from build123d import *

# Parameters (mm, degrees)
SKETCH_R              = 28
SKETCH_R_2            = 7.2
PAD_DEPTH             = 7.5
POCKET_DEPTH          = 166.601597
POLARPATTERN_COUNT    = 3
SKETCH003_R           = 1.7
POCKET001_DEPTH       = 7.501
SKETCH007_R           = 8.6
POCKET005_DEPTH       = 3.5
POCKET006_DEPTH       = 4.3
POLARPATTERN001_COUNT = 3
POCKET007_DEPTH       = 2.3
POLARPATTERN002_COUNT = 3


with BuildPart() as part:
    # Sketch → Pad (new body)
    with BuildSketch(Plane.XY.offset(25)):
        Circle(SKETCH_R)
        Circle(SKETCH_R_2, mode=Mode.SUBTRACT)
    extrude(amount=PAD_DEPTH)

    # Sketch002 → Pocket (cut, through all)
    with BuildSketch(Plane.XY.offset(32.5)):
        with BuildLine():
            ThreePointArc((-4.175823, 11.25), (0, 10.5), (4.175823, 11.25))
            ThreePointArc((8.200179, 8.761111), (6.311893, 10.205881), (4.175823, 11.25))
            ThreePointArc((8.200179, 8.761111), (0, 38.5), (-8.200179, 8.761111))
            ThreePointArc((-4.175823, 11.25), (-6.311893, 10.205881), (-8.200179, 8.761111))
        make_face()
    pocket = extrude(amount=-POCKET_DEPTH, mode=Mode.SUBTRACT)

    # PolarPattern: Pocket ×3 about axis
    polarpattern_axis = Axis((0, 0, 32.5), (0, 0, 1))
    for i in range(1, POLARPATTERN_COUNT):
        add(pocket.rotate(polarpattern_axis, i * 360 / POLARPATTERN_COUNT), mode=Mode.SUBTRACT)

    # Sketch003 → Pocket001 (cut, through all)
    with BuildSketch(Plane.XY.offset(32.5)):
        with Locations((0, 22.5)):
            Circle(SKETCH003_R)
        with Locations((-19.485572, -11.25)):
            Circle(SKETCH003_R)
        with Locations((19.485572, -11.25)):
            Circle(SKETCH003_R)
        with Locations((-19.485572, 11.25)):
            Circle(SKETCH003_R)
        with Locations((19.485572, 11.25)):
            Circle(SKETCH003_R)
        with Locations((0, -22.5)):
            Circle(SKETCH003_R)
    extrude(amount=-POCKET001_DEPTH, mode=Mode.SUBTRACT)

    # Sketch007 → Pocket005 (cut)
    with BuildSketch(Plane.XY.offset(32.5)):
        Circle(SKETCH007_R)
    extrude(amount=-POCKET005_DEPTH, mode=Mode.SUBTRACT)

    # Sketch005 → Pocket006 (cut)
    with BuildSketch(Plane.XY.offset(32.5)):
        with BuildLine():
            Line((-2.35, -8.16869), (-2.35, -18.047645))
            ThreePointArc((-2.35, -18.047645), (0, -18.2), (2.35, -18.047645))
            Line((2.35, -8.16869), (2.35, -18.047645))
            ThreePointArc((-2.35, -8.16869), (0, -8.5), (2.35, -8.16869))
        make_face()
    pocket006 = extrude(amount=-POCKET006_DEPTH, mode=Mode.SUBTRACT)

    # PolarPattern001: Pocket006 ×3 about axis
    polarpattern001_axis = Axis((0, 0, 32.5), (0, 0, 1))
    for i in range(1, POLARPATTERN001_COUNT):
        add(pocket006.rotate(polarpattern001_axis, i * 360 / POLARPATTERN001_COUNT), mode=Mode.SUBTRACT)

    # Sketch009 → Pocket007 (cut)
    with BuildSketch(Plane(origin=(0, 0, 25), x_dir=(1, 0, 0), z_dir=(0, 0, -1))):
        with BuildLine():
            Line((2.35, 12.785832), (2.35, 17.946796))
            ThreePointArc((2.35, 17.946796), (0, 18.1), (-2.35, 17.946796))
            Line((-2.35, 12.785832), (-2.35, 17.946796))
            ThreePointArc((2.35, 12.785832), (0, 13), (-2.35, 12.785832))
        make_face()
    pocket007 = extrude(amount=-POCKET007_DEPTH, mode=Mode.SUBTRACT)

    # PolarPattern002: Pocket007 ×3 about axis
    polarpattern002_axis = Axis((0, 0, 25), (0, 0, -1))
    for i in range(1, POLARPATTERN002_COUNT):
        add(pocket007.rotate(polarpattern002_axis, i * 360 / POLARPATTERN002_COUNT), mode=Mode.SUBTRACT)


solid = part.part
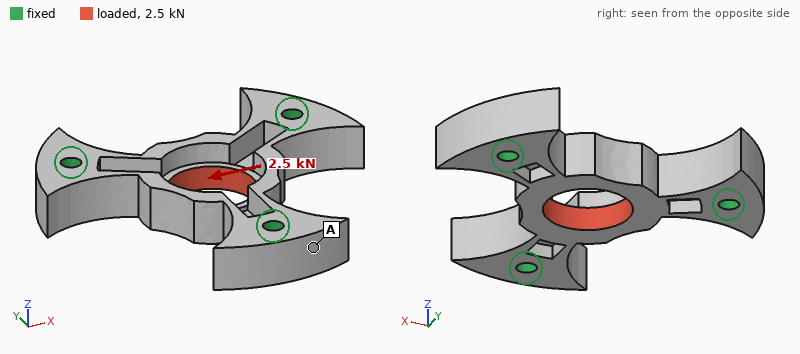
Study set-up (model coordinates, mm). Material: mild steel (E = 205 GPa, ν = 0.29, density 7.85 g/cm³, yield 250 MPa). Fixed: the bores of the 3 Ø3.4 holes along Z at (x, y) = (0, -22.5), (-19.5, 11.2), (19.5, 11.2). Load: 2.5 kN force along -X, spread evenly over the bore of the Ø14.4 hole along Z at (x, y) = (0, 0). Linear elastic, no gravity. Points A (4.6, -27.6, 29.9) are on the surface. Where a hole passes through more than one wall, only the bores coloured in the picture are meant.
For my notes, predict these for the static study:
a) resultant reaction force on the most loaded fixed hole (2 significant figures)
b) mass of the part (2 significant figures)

1.1 kN
42 g
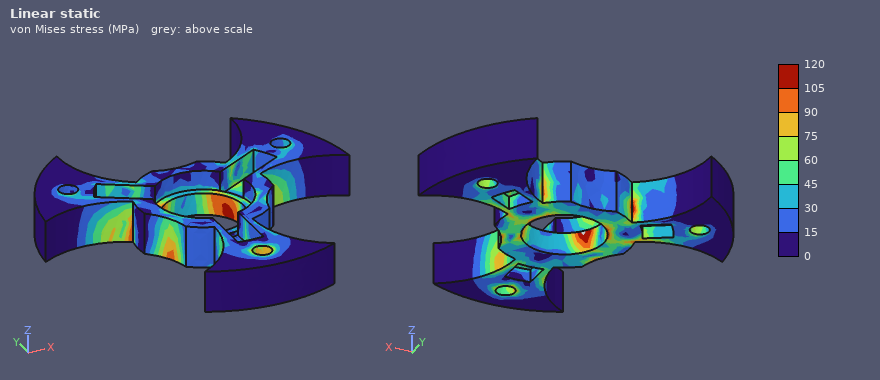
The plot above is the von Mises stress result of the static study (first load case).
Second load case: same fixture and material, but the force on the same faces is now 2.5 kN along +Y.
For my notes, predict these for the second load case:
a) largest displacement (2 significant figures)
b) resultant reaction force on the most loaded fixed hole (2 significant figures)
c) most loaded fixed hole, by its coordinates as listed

15 µm
1.2 kN
(0, -22.5)
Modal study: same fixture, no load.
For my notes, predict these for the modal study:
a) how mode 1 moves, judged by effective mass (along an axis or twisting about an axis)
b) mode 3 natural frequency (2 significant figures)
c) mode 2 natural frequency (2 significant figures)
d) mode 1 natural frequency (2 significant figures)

along Z
20 kHz
20 kHz
19 kHz
